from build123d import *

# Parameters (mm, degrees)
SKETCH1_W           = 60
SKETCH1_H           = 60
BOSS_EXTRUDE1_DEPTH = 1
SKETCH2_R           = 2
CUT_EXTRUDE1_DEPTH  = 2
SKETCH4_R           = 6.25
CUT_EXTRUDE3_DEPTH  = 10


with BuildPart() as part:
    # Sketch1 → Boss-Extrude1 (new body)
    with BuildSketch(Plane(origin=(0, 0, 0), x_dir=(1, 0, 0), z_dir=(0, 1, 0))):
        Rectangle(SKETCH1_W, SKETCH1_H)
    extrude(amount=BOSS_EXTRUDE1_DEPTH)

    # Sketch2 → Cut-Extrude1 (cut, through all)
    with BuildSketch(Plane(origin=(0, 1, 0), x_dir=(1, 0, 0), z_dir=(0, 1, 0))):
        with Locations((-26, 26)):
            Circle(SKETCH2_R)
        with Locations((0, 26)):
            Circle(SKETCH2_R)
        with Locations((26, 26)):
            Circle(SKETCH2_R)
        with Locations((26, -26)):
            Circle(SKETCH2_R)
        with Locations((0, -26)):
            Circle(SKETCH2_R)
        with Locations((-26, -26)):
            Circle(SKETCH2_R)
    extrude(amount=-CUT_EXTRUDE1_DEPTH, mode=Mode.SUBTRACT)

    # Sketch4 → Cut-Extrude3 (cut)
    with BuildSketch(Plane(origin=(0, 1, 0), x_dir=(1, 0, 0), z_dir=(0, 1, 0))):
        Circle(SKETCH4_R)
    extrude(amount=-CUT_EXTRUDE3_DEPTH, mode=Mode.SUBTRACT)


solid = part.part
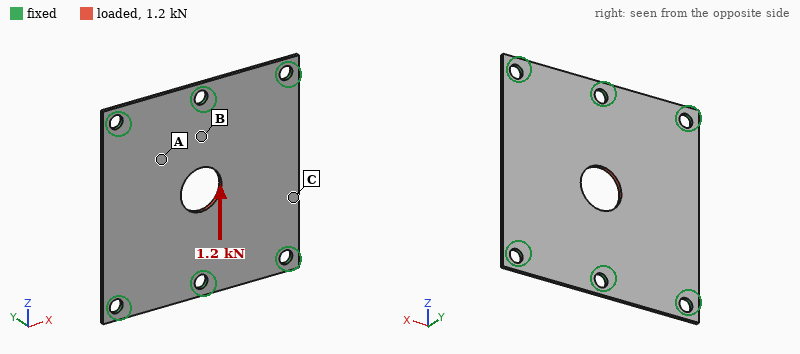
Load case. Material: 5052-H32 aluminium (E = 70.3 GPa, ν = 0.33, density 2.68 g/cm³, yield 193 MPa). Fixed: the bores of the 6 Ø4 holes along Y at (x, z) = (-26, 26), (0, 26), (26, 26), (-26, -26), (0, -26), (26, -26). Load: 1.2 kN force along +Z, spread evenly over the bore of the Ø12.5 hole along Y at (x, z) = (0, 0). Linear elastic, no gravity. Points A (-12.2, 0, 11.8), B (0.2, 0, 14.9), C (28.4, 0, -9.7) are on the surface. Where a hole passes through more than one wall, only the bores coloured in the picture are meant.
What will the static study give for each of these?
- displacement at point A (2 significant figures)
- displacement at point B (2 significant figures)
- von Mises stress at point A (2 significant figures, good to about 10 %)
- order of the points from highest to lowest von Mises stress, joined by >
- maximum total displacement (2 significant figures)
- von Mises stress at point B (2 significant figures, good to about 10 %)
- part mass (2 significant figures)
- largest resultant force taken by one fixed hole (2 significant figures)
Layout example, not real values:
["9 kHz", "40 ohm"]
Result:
["3.8 µm", "4.3 µm", "12 MPa", "B > A > C", "8.3 µm", "27 MPa", "9.1 g", "330 N"]
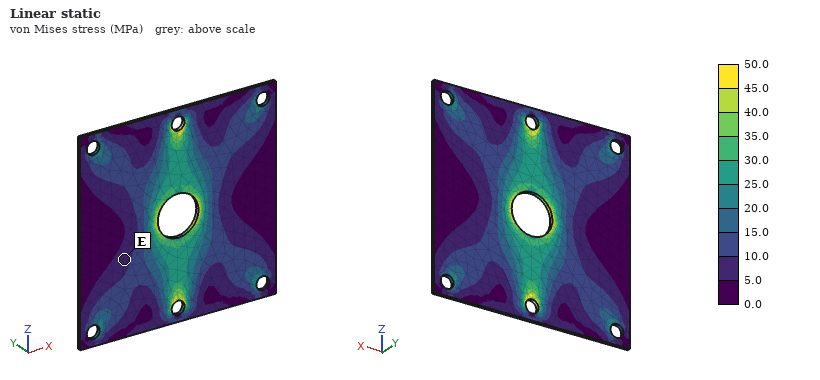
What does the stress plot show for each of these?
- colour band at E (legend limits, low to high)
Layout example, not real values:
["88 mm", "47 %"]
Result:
["5.0 to 10.0 MPa"]
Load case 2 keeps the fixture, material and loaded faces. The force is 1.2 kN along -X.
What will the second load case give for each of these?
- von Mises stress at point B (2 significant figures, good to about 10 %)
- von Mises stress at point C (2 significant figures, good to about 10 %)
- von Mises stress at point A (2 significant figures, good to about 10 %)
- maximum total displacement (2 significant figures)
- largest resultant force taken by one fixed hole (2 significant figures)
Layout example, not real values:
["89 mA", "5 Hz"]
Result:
["18 MPa", "7.5 MPa", "22 MPa", "12 µm", "260 N"]
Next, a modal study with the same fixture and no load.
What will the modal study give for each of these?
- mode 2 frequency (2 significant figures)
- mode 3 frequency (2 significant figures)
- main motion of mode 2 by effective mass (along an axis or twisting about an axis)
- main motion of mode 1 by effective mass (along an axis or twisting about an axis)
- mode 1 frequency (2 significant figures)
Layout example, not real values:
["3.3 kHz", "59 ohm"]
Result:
["2400 Hz", "3600 Hz", "twisting about Z", "along Y", "2000 Hz"]
